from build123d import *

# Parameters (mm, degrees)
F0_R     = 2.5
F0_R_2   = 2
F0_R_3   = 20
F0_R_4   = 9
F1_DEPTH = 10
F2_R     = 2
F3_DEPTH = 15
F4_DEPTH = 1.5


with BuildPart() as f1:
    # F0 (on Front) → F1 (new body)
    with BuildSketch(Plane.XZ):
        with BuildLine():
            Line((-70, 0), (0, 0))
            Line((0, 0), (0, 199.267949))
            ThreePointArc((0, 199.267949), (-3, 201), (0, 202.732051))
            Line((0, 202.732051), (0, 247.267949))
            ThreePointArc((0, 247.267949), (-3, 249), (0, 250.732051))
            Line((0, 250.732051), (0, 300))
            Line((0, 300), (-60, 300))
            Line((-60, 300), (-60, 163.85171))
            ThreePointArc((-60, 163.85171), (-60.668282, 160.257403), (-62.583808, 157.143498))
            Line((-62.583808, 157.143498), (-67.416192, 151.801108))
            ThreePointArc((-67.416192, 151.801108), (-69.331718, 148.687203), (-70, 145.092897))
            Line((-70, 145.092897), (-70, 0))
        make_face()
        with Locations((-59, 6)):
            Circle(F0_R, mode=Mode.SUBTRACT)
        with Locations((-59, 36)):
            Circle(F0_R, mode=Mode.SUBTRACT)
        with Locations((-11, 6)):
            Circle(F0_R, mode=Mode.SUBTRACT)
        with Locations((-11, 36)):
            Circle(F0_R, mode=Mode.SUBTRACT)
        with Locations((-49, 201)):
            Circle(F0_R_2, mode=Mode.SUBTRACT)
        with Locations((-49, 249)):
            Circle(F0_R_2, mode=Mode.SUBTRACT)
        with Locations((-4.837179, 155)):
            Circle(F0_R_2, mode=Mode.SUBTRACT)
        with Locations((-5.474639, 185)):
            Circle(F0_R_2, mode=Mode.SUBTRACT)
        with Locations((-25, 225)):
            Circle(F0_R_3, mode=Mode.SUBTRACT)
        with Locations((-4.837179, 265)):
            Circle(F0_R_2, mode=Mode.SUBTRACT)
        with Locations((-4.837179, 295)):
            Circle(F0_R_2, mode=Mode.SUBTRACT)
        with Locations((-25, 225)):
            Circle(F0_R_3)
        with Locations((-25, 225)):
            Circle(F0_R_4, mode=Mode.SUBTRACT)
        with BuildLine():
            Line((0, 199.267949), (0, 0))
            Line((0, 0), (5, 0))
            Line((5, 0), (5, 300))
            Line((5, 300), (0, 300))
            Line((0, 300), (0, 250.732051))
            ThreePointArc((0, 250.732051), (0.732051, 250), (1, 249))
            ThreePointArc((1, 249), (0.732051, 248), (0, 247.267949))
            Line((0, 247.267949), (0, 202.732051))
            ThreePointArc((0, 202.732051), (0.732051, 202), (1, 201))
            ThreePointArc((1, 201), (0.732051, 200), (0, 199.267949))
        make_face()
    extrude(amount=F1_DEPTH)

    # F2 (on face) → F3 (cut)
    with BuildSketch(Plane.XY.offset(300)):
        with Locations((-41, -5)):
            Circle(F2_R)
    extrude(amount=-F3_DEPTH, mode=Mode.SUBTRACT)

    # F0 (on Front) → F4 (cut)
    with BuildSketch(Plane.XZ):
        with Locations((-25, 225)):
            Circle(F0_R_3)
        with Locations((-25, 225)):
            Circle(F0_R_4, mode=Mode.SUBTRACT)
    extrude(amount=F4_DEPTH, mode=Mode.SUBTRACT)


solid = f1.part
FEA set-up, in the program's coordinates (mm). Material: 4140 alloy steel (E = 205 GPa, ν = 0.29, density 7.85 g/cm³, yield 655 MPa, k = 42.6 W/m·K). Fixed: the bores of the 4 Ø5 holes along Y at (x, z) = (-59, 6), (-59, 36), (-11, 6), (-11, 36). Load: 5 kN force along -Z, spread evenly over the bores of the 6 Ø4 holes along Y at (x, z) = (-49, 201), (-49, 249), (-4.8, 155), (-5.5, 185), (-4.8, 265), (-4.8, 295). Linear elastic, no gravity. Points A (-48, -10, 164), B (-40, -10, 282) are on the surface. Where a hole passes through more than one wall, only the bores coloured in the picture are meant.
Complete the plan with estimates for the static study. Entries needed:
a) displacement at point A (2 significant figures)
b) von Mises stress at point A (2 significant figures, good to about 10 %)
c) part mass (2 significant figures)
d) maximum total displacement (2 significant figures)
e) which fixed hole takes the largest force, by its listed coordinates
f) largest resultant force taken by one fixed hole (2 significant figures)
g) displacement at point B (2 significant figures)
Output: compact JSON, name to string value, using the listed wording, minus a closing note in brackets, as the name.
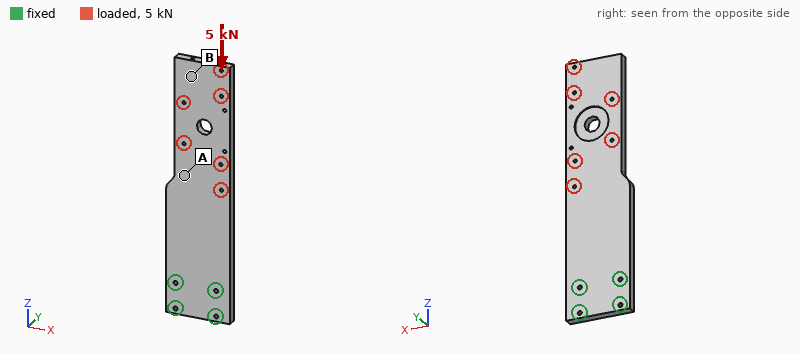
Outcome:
{"displacement at point A": "8.5 µm", "von Mises stress at point A": "4.4 MPa", "part mass": "1.6 kg", "maximum total displacement": "32 µm", "which fixed hole takes the largest force, by its listed coordinates": "(-11, 36)", "largest resultant force taken by one fixed hole": "3.1 kN", "displacement at point B": "26 µm"}
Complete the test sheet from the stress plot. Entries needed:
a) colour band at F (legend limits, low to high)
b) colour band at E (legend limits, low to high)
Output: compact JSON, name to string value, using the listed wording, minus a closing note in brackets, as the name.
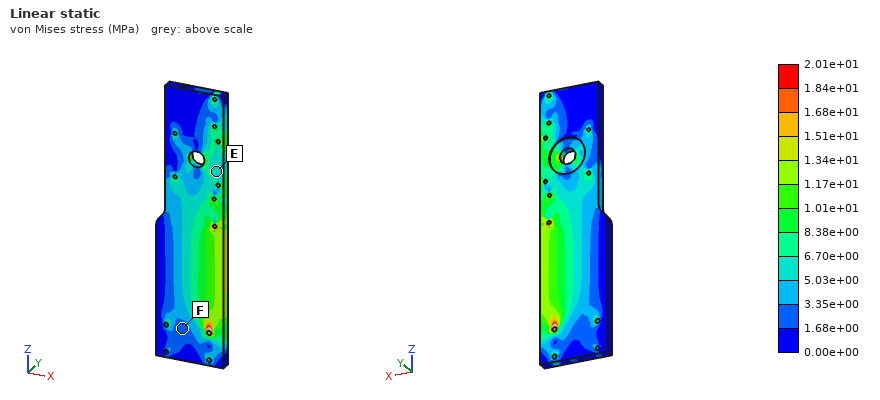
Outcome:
{"colour band at F": "1.68e+00 to 3.35e+00 MPa", "colour band at E": "5.03e+00 to 6.70e+00 MPa"}
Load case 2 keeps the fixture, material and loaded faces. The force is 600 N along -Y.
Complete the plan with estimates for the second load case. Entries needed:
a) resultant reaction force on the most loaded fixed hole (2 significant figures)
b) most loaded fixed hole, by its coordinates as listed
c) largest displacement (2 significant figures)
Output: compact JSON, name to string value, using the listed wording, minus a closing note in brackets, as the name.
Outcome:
{"resultant reaction force on the most loaded fixed hole": "1.4 kN", "most loaded fixed hole, by its coordinates as listed": "(-11, 36)", "largest displacement": "1.9 mm"}
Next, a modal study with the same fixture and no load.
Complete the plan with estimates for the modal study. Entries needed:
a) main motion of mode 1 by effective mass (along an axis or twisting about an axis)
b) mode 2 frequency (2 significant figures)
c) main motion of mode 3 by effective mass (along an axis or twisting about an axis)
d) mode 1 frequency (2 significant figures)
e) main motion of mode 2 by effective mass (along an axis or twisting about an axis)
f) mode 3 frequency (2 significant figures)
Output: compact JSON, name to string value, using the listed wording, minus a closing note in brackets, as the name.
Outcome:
{"main motion of mode 1 by effective mass": "along Y", "mode 2 frequency": "710 Hz", "main motion of mode 3 by effective mass": "along X", "mode 1 frequency": "130 Hz", "main motion of mode 2 by effective mass": "along Y", "mode 3 frequency": "860 Hz"}
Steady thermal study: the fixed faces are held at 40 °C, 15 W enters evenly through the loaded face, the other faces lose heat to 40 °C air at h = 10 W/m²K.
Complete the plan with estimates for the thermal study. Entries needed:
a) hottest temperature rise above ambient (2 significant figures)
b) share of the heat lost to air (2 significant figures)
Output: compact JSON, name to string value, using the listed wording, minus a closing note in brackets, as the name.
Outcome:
{"hottest temperature rise above ambient": "44 K", "share of the heat lost to air": "66 %"}
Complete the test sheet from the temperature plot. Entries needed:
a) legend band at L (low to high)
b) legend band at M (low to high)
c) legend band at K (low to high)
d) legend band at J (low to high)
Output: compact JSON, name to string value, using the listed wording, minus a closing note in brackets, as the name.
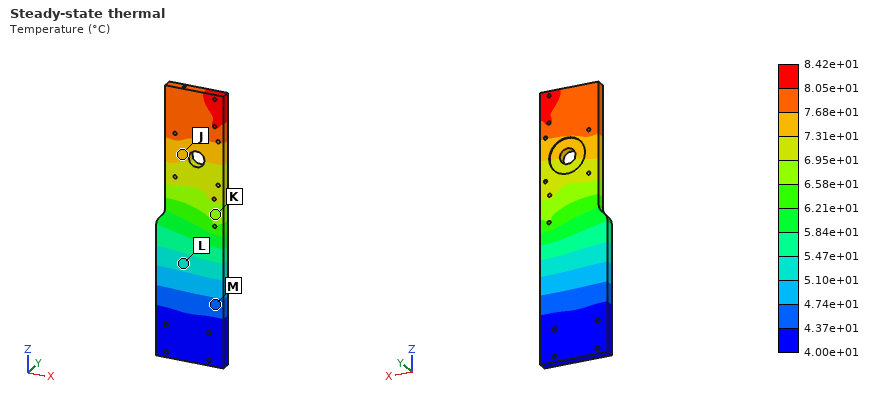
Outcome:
{"legend band at L": "5.10e+01 to 5.47e+01 °C", "legend band at M": "4.37e+01 to 4.74e+01 °C", "legend band at K": "6.58e+01 to 6.95e+01 °C", "legend band at J": "7.31e+01 to 7.68e+01 °C"}
